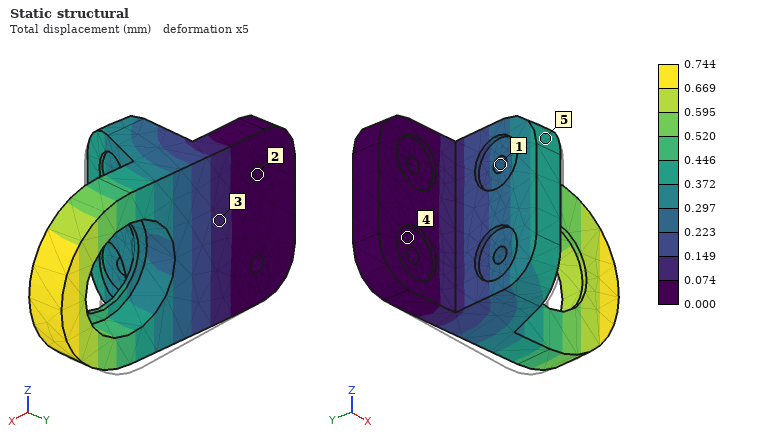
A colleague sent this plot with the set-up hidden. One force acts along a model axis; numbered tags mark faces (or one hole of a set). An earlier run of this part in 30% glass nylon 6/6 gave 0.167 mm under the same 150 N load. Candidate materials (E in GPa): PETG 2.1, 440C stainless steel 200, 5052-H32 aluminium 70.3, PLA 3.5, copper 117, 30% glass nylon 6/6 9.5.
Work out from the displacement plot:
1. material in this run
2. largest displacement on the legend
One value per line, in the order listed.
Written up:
PETG
0.744 mm
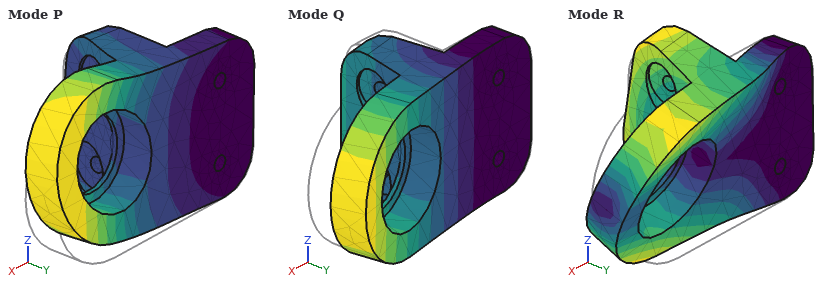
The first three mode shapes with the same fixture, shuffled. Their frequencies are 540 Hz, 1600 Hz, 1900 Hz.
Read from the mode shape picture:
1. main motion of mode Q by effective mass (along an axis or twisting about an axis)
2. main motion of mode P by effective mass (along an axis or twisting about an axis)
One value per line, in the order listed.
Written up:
along Y
along Z
